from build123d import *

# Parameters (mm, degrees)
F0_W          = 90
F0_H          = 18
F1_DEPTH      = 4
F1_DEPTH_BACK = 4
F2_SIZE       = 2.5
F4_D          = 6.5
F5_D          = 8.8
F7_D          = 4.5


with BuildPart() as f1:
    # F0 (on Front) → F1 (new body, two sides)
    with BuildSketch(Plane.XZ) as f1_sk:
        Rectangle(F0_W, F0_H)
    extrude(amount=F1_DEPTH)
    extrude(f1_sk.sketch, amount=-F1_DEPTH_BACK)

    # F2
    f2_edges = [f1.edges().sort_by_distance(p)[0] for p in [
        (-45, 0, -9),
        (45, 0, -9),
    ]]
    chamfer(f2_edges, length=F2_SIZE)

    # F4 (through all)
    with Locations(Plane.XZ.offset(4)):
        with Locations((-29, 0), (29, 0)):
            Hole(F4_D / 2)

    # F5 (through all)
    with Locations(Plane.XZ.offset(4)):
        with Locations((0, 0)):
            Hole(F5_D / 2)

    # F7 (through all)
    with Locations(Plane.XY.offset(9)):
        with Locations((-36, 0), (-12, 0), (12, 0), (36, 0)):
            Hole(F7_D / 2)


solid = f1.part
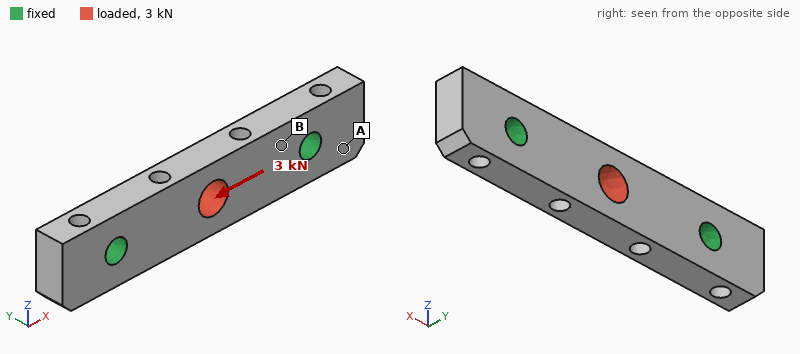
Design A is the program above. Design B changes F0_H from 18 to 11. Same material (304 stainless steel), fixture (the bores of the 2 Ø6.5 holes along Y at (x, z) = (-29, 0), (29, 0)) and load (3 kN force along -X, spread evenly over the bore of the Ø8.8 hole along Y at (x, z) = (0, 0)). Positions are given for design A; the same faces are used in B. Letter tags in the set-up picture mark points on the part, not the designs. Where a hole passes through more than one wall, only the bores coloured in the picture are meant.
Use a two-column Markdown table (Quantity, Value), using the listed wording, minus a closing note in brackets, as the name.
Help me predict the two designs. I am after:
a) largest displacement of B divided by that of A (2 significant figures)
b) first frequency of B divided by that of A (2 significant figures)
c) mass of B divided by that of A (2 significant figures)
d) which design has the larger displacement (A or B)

| Quantity | Value |
|---|---|
| largest displacement of B divided by that of A | 1.6 |
| first frequency of B divided by that of A | 1.0 |
| mass of B divided by that of A | 0.57 |
| which design has the larger displacement | B |
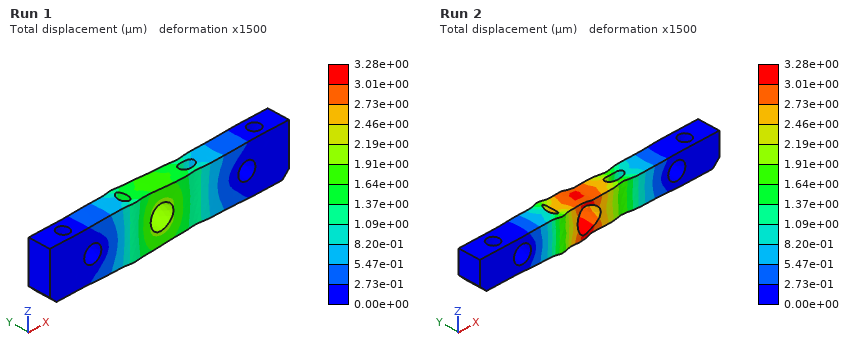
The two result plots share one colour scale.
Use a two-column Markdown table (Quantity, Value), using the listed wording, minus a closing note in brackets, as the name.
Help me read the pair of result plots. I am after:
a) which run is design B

| Quantity | Value |
|---|---|
| which run is design B | Run 2 |
